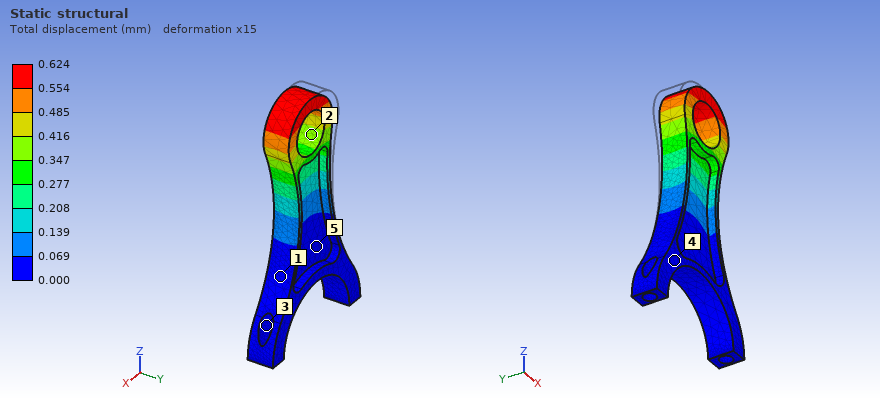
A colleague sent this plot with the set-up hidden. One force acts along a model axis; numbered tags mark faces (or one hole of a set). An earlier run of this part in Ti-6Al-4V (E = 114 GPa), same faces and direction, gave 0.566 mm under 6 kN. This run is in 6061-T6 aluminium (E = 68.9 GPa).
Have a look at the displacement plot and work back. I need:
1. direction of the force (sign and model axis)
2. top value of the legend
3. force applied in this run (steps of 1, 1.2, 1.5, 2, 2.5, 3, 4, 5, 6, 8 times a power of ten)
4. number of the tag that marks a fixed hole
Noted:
+X
0.624 mm
4 kN
3
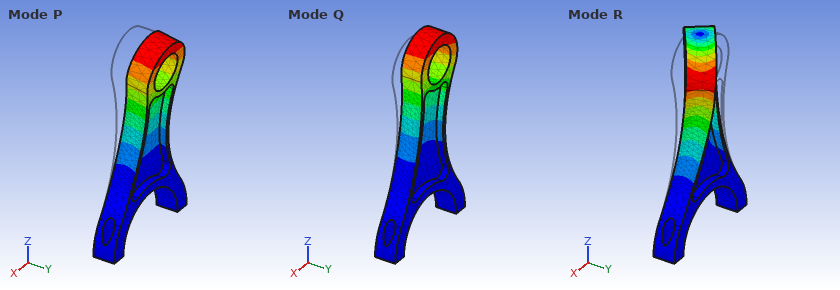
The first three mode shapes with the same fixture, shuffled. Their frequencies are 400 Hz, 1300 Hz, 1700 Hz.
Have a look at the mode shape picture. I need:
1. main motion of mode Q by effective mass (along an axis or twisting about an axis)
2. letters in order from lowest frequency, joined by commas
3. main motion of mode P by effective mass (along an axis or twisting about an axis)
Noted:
along X
P, R, Q
along Y
